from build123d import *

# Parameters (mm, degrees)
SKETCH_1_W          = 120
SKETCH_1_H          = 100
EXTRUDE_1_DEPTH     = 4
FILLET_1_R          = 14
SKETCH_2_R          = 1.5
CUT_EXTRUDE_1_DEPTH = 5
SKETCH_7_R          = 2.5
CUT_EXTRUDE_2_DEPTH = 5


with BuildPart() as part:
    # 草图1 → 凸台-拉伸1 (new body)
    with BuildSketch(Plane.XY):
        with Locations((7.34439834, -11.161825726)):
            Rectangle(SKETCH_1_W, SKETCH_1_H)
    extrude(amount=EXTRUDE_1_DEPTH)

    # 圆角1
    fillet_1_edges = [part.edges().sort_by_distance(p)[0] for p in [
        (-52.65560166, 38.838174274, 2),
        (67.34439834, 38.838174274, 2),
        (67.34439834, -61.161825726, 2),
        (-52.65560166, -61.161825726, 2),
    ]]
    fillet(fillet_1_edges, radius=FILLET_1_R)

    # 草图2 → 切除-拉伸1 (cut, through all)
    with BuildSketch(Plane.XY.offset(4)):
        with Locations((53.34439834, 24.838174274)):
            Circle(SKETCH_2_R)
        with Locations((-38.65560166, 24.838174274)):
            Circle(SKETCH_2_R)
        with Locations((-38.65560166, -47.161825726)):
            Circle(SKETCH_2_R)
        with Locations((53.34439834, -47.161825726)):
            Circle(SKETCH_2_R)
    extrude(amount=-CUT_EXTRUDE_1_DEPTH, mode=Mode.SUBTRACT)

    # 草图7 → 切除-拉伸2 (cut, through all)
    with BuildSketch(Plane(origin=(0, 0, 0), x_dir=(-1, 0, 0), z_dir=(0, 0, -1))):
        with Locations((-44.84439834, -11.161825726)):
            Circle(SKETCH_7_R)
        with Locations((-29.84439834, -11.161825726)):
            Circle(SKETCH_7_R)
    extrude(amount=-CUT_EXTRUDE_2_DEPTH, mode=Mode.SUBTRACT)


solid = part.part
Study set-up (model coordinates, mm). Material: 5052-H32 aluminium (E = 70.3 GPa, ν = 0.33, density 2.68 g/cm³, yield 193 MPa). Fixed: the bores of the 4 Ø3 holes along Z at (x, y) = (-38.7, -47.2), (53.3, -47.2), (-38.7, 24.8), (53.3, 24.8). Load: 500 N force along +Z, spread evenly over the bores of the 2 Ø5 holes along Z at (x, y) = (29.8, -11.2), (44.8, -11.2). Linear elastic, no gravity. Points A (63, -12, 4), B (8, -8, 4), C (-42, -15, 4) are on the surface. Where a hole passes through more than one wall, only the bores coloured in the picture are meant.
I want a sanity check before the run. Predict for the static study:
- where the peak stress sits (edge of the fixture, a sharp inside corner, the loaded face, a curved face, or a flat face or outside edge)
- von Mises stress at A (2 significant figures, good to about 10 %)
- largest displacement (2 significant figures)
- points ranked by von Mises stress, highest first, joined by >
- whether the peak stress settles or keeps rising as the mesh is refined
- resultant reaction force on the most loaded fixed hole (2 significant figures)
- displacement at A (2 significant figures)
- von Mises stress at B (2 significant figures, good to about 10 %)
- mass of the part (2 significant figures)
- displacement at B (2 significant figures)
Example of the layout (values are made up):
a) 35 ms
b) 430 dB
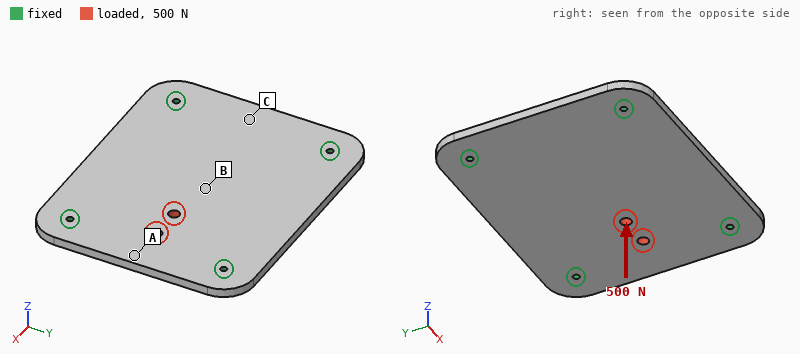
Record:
a) edge of the fixture
b) 22 MPa
c) 91 µm
d) A > B > C
e) keeps rising
f) 210 N
g) 46 µm
h) 12 MPa
i) 130 g
j) 66 µm
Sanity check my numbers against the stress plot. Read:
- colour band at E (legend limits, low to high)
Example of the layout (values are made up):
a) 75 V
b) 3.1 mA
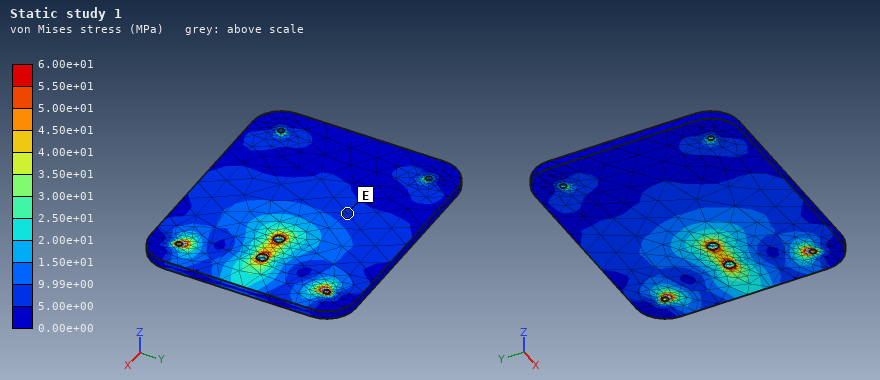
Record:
a) 5.00e+00 to 9.99e+00 MPa
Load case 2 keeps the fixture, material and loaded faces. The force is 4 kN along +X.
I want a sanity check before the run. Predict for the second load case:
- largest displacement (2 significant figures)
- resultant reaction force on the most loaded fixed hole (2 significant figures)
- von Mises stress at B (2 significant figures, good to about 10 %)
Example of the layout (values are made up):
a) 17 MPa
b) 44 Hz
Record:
a) 17 µm
b) 1.2 kN
c) 13 MPa
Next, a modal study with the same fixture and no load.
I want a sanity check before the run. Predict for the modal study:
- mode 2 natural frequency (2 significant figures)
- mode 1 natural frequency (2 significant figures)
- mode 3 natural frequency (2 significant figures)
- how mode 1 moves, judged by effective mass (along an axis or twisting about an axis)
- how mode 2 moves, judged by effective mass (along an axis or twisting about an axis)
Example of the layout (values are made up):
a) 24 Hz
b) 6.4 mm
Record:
a) 2600 Hz
b) 1900 Hz
c) 3200 Hz
d) along Z
e) twisting about X
